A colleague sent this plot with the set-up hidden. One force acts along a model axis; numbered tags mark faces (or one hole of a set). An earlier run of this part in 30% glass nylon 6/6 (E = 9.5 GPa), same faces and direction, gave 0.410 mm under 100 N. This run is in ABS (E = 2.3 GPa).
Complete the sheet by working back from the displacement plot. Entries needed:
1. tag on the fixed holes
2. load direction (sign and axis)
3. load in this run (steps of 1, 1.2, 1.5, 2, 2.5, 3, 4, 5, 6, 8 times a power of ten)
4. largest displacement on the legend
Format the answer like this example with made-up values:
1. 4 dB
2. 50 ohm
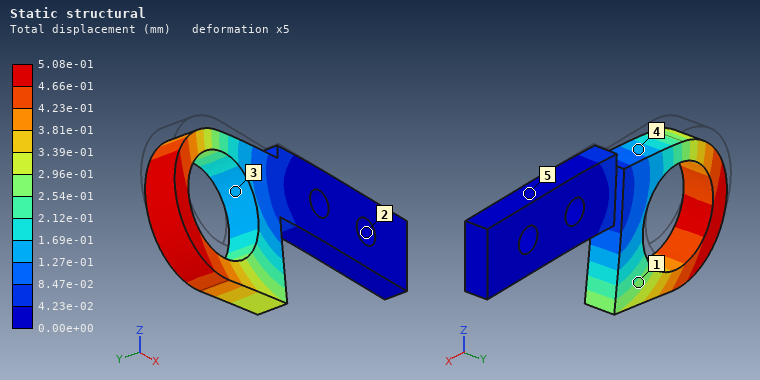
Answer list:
1. 2
2. -Z
3. 30 N
4. 5.08e-01 mm
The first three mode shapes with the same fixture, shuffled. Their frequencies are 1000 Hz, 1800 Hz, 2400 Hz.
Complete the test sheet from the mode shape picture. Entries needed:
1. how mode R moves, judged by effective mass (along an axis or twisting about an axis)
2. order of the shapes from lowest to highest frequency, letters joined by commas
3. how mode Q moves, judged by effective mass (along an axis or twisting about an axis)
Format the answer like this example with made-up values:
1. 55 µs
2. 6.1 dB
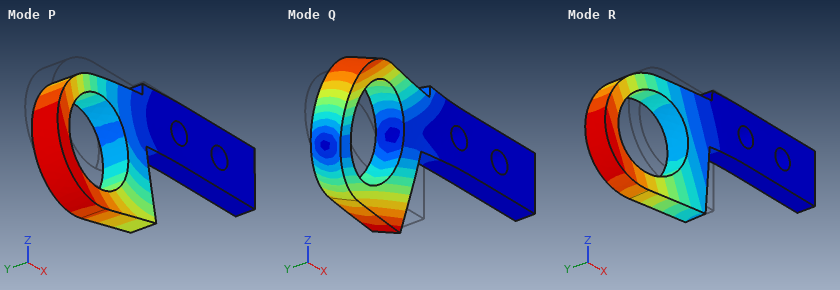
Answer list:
1. along Y
2. R, P, Q
3. twisting about X
